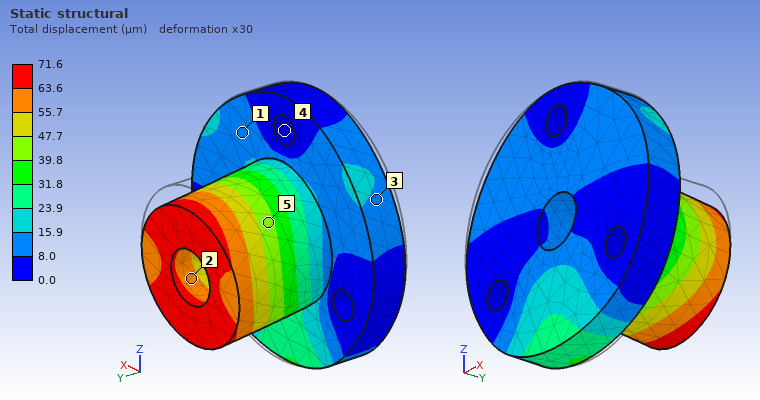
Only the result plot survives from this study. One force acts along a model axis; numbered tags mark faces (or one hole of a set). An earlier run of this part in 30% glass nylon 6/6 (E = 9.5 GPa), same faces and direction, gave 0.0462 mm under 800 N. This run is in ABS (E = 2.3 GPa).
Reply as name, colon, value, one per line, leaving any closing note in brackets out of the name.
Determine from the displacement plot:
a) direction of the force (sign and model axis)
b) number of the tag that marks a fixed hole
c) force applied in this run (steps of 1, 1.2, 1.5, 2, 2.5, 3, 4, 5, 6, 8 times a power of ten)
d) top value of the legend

direction of the force: -Z
number of the tag that marks a fixed hole: 4
force applied in this run: 300 N
top value of the legend: 71.6 µm
